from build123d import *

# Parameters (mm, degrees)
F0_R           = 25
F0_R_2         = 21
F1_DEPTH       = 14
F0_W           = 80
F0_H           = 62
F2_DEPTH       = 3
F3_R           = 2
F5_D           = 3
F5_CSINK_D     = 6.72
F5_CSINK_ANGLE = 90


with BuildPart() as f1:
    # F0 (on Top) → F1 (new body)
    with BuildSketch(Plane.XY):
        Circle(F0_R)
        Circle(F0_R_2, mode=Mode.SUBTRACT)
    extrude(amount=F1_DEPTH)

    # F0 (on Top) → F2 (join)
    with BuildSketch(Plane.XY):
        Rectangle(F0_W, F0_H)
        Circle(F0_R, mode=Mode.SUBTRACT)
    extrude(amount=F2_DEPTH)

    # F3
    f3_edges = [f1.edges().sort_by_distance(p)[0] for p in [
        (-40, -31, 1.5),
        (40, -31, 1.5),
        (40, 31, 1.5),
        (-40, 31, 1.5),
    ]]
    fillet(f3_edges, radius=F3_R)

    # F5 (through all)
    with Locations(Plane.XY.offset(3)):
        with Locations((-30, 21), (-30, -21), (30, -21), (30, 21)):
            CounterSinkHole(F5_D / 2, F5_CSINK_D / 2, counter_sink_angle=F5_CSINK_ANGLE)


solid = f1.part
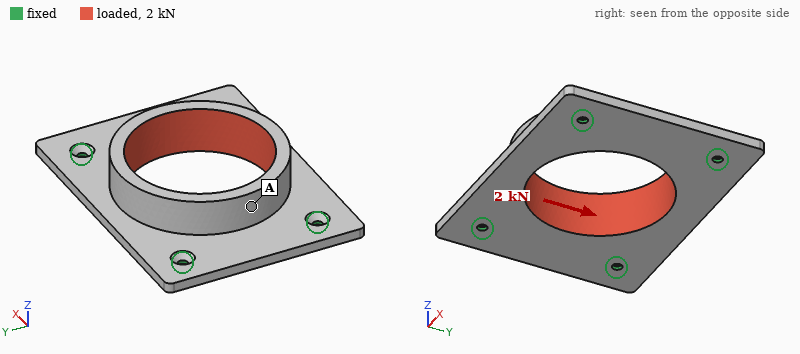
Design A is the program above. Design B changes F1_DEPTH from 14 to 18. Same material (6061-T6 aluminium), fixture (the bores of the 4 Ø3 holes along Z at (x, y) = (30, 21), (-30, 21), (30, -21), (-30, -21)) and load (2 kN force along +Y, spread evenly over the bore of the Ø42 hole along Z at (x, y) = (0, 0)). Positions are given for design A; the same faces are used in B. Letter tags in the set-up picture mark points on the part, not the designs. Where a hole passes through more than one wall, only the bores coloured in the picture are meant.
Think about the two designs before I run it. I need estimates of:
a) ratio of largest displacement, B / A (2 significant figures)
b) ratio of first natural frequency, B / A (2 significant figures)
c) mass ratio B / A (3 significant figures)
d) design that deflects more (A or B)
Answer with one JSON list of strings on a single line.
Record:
["1.3", "0.96", "1.14", "B"]
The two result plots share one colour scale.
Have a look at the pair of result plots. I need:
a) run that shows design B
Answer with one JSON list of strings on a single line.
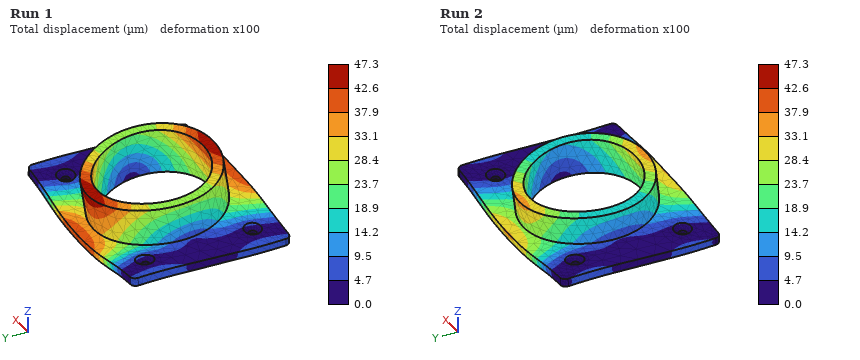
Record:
["Run 1"]
